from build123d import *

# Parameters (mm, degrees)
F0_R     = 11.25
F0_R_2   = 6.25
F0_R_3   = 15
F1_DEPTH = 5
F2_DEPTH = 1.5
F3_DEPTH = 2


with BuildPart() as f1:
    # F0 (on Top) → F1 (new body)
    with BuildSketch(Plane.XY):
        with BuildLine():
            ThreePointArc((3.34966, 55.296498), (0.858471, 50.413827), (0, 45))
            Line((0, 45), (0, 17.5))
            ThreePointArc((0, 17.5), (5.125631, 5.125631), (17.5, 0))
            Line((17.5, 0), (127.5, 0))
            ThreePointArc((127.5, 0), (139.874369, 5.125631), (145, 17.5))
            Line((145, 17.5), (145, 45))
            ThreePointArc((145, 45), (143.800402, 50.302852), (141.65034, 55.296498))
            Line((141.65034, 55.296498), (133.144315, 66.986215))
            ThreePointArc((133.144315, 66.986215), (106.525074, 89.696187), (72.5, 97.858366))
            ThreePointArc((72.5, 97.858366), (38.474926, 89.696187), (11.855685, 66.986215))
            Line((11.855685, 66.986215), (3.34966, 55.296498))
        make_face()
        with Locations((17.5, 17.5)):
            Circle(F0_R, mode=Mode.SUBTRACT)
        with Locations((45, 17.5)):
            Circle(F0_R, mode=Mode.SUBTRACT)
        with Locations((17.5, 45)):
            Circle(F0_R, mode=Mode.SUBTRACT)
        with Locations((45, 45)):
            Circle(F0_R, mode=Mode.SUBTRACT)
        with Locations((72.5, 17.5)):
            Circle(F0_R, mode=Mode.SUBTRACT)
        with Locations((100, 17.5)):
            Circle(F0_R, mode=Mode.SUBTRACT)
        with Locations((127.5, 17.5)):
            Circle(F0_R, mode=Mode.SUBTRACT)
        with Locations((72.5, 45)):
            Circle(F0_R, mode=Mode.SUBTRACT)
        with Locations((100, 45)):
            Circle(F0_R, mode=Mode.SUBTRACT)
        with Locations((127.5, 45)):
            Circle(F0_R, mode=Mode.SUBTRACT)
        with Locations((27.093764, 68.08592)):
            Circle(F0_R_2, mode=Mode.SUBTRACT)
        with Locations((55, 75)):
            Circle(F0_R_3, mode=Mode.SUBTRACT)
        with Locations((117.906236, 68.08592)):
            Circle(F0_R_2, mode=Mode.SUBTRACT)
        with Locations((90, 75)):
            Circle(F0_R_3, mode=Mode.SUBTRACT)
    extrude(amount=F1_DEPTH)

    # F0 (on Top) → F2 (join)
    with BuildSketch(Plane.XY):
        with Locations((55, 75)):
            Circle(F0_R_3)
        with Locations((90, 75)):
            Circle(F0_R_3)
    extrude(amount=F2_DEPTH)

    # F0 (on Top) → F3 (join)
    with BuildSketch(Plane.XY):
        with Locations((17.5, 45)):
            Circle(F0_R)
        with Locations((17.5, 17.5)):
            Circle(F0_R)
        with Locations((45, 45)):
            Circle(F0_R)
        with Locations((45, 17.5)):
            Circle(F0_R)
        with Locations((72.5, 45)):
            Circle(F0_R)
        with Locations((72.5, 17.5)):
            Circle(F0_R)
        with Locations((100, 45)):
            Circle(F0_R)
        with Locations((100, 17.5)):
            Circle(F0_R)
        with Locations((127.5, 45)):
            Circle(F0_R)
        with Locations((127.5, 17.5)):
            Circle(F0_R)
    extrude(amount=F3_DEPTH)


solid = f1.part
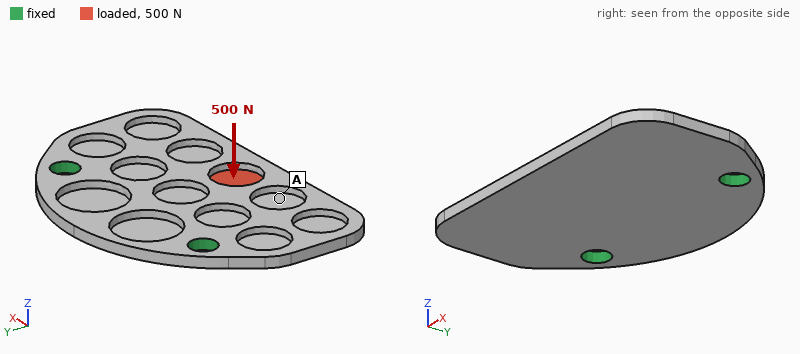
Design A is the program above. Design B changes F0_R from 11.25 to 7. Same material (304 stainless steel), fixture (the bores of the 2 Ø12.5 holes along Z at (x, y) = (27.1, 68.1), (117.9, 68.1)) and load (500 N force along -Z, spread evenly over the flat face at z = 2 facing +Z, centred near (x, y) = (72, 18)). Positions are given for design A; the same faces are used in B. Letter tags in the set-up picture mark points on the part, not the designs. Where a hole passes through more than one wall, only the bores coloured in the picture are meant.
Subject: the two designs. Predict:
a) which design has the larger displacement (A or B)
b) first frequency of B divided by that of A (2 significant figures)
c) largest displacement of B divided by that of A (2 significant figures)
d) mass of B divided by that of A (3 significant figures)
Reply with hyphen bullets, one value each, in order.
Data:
- A
- 1.1
- 0.71
- 1.17
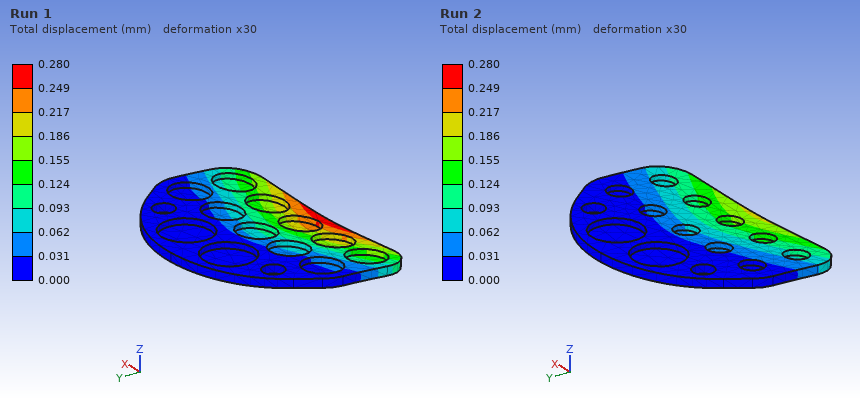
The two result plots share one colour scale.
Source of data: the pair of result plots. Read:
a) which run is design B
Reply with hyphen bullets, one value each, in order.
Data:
- Run 2
